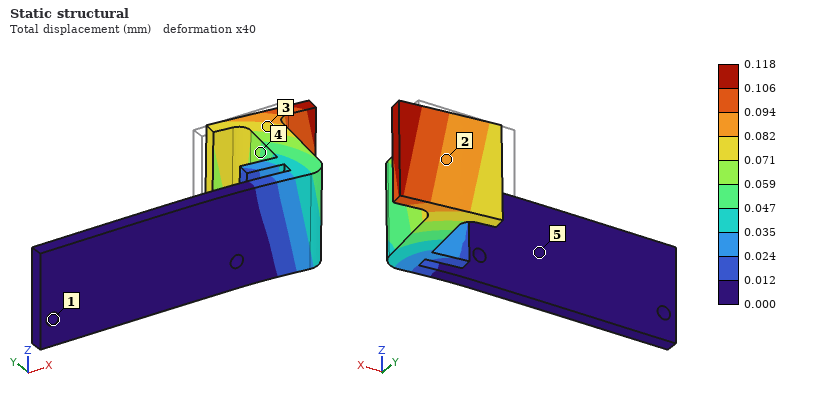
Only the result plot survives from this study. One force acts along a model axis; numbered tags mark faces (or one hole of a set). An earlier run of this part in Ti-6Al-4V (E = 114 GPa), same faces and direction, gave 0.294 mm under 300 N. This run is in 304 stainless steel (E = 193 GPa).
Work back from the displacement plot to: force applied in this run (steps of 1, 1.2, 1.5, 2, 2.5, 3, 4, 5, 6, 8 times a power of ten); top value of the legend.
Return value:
200 N
0.118 mm
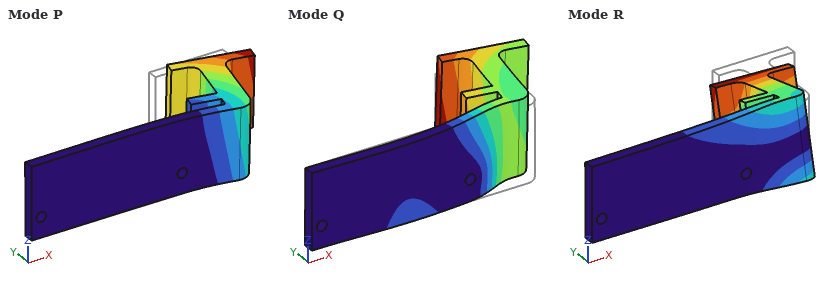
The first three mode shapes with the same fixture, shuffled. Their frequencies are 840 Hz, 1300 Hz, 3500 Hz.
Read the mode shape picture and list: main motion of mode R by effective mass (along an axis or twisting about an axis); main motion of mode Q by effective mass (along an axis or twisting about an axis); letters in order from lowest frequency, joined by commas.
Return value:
along Z
along Y
P, R, Q
